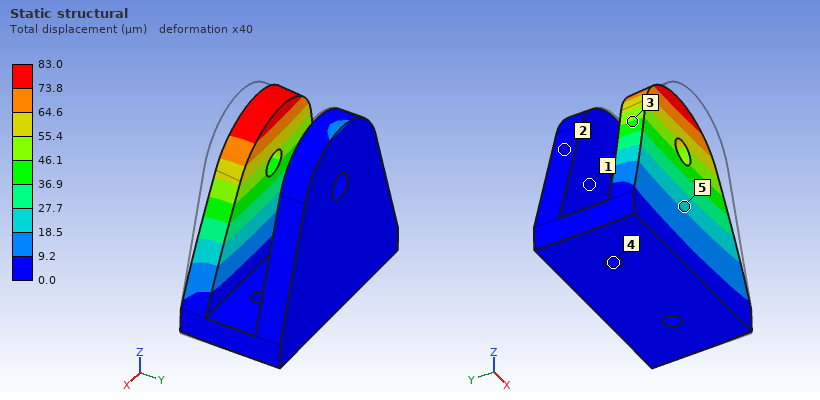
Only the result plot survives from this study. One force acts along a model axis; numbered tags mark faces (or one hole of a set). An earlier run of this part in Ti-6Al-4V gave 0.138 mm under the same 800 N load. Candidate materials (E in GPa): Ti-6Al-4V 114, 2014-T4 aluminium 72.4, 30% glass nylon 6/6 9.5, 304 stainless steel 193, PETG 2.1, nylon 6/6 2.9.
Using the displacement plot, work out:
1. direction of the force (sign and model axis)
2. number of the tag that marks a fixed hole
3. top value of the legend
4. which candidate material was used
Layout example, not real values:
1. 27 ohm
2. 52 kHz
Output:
1. +Y
2. 4
3. 83.0 µm
4. 304 stainless steel
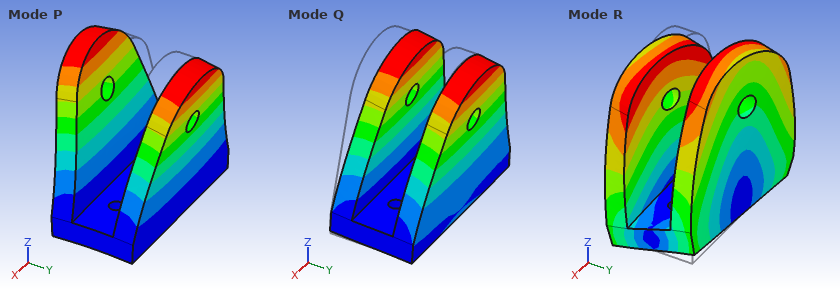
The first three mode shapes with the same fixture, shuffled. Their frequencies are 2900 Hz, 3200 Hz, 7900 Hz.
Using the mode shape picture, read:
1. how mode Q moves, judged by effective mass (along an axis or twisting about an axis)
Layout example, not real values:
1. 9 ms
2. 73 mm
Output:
1. along Y
